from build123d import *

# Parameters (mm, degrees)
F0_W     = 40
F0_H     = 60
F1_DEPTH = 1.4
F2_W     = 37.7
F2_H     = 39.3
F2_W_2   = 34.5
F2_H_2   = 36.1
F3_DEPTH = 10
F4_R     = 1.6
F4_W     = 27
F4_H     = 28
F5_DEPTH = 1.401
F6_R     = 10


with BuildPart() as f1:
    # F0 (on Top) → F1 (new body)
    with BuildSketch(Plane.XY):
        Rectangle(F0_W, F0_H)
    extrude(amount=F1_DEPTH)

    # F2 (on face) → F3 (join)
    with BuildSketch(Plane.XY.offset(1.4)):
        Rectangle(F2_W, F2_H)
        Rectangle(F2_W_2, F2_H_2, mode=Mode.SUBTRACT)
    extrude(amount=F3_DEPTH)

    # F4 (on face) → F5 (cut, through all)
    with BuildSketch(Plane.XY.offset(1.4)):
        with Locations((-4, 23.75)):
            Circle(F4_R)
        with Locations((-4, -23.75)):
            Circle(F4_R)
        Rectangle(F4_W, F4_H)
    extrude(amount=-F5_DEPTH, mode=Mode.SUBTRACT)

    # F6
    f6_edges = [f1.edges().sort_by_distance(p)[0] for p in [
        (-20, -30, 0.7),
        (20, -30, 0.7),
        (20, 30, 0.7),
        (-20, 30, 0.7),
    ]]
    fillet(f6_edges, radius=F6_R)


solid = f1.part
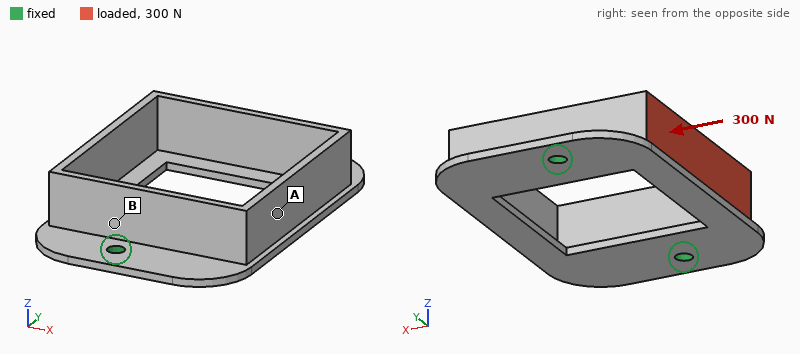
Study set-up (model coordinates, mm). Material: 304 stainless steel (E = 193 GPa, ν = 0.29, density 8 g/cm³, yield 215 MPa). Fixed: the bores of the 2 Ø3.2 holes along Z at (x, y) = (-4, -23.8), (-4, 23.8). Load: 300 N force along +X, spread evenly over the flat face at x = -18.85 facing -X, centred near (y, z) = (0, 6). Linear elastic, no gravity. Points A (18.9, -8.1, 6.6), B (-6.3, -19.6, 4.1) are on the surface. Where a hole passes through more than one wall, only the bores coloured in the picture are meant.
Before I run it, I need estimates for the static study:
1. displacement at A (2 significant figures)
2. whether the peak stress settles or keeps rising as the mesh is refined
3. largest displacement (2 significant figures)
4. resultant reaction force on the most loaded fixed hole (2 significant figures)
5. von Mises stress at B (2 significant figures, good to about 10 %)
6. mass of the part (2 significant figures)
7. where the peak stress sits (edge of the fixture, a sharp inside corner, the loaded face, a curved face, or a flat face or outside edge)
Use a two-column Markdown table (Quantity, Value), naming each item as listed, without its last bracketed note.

| Quantity | Value |
|---|---|
| displacement at A | 42 µm |
| whether the peak stress settles or keeps rising as the mesh is refined | keeps rising |
| largest displacement | 67 µm |
| resultant reaction force on the most loaded fixed hole | 160 N |
| von Mises stress at B | 21 MPa |
| mass of the part | 36 g |
| where the peak stress sits | edge of the fixture |
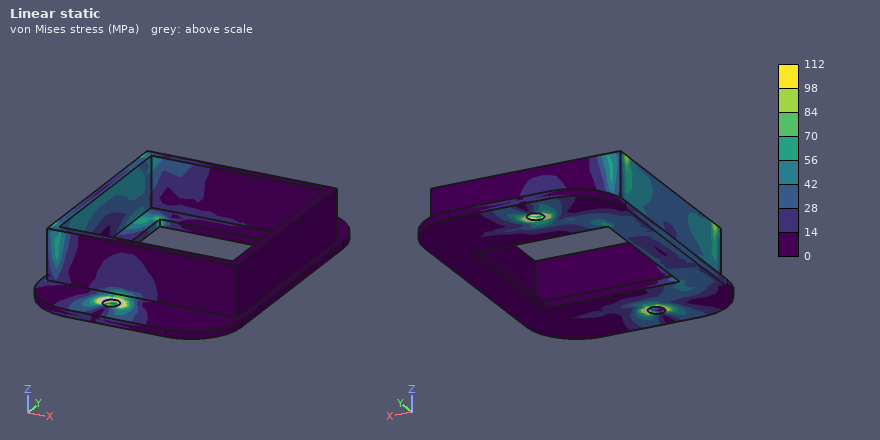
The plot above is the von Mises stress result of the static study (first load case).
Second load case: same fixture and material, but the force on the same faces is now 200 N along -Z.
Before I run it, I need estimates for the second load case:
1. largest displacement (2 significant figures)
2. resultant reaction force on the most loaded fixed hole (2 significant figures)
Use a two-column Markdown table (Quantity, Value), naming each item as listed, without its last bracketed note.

| Quantity | Value |
|---|---|
| largest displacement | 75 µm |
| resultant reaction force on the most loaded fixed hole | 110 N |
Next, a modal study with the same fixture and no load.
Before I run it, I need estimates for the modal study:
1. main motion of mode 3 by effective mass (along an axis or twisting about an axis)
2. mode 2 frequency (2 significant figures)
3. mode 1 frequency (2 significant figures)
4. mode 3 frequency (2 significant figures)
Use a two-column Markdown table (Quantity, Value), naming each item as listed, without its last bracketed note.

| Quantity | Value |
|---|---|
| main motion of mode 3 by effective mass | along Z |
| mode 2 frequency | 3200 Hz |
| mode 1 frequency | 1700 Hz |
| mode 3 frequency | 6200 Hz |
